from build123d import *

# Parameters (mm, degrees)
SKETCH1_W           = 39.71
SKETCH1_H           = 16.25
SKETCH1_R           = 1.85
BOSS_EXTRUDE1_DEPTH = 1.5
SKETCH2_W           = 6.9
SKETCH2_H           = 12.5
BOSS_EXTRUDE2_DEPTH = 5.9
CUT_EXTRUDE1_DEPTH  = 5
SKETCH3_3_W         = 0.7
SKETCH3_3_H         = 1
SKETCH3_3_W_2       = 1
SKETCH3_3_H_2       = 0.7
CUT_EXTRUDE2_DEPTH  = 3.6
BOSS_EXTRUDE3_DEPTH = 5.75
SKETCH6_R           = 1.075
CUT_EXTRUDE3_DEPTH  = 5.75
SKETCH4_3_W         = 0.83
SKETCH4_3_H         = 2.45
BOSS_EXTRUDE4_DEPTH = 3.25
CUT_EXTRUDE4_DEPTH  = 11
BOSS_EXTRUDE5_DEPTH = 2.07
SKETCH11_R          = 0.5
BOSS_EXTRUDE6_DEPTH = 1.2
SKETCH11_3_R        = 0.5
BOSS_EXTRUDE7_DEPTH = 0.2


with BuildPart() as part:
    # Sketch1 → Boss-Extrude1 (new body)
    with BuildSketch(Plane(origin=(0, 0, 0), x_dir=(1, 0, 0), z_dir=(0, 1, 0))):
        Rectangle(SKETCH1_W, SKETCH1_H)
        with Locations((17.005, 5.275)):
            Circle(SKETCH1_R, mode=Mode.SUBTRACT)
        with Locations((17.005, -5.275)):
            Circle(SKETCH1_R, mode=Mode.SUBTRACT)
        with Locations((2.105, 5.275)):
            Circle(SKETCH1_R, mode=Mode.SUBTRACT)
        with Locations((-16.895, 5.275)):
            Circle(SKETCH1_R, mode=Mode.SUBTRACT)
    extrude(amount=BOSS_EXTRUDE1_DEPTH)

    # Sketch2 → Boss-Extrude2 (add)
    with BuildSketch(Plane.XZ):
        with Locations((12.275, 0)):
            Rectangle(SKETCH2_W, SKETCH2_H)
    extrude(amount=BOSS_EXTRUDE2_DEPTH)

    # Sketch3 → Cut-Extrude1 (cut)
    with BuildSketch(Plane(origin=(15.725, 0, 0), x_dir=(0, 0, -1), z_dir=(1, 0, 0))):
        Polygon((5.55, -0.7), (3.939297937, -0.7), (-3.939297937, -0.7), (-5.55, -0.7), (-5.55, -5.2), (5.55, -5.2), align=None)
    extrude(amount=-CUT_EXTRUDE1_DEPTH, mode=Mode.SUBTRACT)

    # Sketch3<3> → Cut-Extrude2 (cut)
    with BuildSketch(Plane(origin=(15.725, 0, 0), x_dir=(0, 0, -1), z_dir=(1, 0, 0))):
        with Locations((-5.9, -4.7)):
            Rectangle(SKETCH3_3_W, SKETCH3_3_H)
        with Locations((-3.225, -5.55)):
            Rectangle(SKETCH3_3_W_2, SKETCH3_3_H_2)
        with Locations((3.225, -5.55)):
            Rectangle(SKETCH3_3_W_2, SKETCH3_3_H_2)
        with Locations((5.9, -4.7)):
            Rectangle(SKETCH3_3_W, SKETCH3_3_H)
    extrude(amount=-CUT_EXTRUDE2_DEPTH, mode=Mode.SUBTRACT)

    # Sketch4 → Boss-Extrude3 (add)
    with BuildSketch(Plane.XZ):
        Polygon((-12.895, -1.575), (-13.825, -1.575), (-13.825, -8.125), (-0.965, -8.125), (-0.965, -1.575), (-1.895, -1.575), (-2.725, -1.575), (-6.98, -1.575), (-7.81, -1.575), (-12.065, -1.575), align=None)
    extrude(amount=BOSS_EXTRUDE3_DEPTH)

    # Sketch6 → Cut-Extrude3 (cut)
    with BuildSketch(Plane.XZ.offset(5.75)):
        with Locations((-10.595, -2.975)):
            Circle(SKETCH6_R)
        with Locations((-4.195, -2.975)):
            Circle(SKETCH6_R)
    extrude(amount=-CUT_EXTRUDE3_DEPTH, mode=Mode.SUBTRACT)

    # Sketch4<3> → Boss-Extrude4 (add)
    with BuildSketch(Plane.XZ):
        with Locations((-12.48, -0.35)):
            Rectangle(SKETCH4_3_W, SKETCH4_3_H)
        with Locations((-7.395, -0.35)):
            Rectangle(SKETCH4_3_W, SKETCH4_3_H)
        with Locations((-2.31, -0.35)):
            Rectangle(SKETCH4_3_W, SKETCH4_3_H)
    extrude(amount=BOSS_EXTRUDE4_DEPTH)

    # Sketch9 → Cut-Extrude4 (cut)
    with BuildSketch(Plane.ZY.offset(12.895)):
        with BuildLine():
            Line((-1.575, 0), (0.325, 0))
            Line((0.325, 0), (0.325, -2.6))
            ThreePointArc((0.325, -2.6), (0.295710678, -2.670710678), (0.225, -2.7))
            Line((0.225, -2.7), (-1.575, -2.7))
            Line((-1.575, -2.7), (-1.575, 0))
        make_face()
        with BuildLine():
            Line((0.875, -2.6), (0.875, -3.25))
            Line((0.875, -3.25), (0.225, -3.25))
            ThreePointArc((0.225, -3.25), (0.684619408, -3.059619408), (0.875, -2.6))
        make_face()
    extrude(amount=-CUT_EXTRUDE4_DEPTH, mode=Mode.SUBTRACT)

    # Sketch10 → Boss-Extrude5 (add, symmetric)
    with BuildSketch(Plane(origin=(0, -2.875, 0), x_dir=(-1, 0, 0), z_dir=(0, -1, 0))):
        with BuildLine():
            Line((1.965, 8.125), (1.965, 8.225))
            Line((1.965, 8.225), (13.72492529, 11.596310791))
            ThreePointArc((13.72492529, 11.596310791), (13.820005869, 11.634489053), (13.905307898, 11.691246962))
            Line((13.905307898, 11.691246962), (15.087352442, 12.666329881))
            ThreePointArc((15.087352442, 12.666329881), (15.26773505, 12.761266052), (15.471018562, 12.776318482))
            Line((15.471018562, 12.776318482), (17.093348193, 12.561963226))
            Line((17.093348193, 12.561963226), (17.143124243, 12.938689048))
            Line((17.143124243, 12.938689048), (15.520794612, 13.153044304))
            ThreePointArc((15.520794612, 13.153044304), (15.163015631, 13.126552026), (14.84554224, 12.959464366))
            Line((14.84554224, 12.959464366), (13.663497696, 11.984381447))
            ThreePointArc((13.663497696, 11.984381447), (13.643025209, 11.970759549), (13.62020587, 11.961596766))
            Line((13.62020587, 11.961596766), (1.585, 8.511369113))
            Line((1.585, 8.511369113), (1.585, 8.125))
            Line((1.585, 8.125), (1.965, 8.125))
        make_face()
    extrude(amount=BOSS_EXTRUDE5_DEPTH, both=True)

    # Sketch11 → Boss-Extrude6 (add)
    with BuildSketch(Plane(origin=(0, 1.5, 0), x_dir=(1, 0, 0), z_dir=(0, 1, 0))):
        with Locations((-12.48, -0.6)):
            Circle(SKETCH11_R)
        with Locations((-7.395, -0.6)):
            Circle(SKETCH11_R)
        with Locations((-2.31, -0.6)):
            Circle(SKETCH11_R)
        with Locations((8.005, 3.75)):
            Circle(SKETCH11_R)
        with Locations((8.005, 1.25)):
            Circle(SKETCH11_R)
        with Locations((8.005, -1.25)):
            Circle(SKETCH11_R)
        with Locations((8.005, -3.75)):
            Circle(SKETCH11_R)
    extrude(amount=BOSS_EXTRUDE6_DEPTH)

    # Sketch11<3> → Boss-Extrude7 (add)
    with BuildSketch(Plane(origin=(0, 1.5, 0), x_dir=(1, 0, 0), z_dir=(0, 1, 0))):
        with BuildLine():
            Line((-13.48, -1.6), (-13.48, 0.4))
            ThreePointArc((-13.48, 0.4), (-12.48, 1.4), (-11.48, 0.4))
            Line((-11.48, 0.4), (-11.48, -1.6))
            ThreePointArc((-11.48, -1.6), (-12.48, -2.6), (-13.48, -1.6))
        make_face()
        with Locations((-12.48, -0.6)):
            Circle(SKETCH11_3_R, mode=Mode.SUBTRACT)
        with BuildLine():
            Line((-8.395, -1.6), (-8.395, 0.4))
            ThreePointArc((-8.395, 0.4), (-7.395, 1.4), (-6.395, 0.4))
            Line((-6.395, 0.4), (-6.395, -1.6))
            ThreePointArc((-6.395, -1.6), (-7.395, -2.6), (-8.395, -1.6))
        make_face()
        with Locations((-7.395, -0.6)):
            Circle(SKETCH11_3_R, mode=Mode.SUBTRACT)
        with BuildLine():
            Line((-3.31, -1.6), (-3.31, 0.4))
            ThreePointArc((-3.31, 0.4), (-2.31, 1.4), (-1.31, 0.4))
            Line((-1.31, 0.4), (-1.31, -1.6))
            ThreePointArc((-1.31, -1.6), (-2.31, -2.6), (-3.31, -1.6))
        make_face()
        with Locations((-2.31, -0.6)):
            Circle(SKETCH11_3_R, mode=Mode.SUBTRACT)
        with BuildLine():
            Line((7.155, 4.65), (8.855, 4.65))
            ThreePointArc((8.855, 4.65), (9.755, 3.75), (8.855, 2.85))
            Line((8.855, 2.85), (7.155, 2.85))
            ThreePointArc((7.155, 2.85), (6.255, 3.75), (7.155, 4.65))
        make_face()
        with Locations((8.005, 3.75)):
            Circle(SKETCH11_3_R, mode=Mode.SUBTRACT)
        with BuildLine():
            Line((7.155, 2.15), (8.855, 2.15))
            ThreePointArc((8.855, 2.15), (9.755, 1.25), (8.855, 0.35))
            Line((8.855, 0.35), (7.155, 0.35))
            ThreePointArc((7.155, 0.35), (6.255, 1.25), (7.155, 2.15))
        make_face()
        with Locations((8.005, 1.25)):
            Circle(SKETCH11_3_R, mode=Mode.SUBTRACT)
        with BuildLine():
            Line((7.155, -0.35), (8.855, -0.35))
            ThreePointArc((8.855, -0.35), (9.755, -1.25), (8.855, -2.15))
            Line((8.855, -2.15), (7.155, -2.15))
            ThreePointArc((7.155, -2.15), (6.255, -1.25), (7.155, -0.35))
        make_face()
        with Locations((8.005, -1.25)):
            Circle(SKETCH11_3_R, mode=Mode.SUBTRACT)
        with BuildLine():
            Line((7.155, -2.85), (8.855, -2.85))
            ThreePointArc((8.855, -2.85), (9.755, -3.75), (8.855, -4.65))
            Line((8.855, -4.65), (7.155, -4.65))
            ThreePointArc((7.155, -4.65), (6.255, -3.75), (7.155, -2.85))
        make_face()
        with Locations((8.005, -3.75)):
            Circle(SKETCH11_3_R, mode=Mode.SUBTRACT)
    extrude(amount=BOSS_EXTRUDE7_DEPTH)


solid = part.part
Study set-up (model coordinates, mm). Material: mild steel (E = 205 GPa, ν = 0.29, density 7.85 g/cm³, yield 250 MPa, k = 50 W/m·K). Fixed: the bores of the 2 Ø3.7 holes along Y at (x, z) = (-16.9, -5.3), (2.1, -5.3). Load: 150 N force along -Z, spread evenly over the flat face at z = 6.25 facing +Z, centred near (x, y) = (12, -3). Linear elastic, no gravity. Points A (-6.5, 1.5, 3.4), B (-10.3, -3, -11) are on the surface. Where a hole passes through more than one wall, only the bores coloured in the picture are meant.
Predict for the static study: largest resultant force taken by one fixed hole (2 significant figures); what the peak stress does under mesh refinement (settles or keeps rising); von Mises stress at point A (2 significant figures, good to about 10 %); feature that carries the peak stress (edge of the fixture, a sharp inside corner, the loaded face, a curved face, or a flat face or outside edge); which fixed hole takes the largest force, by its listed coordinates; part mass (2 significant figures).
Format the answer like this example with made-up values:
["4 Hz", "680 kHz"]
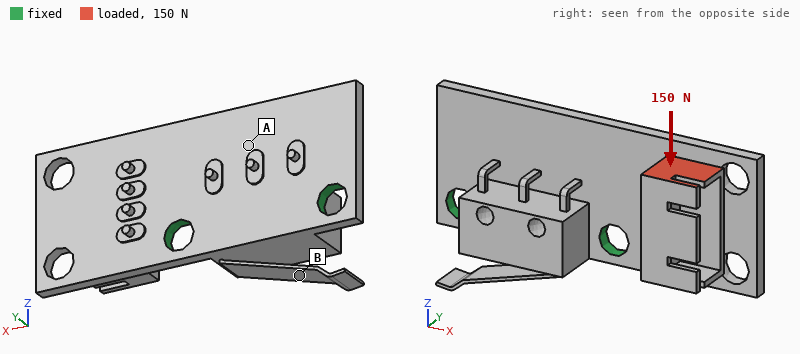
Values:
["210 N", "keeps rising", "25 MPa", "edge of the fixture", "(2.1, -5.3)", "13 g"]
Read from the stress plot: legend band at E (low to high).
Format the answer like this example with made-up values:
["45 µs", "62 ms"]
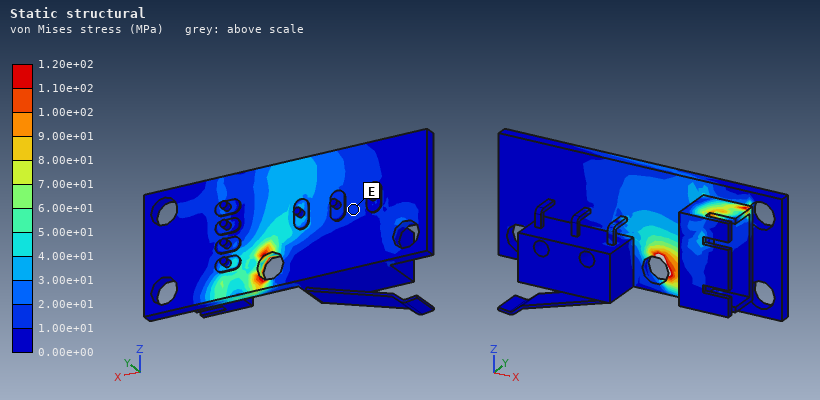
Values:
["1.00e+01 to 2.00e+01 MPa"]
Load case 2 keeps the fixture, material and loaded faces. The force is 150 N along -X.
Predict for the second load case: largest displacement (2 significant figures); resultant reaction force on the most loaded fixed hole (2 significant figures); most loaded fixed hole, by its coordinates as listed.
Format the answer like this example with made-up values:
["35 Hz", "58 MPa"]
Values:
["69 µm", "110 N", "(-16.9, -5.3)"]
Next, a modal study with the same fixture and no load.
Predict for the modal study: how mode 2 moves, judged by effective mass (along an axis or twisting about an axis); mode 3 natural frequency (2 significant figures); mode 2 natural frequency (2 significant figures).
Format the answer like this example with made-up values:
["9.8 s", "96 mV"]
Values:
["along Y", "7000 Hz", "3300 Hz"]
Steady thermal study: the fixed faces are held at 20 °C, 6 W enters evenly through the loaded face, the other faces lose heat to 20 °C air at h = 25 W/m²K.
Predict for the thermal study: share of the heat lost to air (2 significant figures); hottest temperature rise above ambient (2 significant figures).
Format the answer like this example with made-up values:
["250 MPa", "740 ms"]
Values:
["19 %", "85 K"]
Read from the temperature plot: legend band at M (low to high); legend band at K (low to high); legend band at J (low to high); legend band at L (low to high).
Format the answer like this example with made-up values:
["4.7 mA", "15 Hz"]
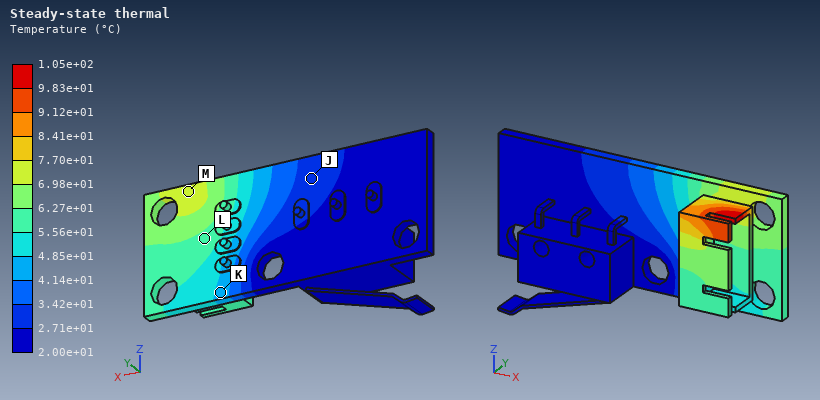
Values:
["6.98e+01 to 7.70e+01 °C", "4.14e+01 to 4.85e+01 °C", "2.71e+01 to 3.42e+01 °C", "5.56e+01 to 6.27e+01 °C"]
